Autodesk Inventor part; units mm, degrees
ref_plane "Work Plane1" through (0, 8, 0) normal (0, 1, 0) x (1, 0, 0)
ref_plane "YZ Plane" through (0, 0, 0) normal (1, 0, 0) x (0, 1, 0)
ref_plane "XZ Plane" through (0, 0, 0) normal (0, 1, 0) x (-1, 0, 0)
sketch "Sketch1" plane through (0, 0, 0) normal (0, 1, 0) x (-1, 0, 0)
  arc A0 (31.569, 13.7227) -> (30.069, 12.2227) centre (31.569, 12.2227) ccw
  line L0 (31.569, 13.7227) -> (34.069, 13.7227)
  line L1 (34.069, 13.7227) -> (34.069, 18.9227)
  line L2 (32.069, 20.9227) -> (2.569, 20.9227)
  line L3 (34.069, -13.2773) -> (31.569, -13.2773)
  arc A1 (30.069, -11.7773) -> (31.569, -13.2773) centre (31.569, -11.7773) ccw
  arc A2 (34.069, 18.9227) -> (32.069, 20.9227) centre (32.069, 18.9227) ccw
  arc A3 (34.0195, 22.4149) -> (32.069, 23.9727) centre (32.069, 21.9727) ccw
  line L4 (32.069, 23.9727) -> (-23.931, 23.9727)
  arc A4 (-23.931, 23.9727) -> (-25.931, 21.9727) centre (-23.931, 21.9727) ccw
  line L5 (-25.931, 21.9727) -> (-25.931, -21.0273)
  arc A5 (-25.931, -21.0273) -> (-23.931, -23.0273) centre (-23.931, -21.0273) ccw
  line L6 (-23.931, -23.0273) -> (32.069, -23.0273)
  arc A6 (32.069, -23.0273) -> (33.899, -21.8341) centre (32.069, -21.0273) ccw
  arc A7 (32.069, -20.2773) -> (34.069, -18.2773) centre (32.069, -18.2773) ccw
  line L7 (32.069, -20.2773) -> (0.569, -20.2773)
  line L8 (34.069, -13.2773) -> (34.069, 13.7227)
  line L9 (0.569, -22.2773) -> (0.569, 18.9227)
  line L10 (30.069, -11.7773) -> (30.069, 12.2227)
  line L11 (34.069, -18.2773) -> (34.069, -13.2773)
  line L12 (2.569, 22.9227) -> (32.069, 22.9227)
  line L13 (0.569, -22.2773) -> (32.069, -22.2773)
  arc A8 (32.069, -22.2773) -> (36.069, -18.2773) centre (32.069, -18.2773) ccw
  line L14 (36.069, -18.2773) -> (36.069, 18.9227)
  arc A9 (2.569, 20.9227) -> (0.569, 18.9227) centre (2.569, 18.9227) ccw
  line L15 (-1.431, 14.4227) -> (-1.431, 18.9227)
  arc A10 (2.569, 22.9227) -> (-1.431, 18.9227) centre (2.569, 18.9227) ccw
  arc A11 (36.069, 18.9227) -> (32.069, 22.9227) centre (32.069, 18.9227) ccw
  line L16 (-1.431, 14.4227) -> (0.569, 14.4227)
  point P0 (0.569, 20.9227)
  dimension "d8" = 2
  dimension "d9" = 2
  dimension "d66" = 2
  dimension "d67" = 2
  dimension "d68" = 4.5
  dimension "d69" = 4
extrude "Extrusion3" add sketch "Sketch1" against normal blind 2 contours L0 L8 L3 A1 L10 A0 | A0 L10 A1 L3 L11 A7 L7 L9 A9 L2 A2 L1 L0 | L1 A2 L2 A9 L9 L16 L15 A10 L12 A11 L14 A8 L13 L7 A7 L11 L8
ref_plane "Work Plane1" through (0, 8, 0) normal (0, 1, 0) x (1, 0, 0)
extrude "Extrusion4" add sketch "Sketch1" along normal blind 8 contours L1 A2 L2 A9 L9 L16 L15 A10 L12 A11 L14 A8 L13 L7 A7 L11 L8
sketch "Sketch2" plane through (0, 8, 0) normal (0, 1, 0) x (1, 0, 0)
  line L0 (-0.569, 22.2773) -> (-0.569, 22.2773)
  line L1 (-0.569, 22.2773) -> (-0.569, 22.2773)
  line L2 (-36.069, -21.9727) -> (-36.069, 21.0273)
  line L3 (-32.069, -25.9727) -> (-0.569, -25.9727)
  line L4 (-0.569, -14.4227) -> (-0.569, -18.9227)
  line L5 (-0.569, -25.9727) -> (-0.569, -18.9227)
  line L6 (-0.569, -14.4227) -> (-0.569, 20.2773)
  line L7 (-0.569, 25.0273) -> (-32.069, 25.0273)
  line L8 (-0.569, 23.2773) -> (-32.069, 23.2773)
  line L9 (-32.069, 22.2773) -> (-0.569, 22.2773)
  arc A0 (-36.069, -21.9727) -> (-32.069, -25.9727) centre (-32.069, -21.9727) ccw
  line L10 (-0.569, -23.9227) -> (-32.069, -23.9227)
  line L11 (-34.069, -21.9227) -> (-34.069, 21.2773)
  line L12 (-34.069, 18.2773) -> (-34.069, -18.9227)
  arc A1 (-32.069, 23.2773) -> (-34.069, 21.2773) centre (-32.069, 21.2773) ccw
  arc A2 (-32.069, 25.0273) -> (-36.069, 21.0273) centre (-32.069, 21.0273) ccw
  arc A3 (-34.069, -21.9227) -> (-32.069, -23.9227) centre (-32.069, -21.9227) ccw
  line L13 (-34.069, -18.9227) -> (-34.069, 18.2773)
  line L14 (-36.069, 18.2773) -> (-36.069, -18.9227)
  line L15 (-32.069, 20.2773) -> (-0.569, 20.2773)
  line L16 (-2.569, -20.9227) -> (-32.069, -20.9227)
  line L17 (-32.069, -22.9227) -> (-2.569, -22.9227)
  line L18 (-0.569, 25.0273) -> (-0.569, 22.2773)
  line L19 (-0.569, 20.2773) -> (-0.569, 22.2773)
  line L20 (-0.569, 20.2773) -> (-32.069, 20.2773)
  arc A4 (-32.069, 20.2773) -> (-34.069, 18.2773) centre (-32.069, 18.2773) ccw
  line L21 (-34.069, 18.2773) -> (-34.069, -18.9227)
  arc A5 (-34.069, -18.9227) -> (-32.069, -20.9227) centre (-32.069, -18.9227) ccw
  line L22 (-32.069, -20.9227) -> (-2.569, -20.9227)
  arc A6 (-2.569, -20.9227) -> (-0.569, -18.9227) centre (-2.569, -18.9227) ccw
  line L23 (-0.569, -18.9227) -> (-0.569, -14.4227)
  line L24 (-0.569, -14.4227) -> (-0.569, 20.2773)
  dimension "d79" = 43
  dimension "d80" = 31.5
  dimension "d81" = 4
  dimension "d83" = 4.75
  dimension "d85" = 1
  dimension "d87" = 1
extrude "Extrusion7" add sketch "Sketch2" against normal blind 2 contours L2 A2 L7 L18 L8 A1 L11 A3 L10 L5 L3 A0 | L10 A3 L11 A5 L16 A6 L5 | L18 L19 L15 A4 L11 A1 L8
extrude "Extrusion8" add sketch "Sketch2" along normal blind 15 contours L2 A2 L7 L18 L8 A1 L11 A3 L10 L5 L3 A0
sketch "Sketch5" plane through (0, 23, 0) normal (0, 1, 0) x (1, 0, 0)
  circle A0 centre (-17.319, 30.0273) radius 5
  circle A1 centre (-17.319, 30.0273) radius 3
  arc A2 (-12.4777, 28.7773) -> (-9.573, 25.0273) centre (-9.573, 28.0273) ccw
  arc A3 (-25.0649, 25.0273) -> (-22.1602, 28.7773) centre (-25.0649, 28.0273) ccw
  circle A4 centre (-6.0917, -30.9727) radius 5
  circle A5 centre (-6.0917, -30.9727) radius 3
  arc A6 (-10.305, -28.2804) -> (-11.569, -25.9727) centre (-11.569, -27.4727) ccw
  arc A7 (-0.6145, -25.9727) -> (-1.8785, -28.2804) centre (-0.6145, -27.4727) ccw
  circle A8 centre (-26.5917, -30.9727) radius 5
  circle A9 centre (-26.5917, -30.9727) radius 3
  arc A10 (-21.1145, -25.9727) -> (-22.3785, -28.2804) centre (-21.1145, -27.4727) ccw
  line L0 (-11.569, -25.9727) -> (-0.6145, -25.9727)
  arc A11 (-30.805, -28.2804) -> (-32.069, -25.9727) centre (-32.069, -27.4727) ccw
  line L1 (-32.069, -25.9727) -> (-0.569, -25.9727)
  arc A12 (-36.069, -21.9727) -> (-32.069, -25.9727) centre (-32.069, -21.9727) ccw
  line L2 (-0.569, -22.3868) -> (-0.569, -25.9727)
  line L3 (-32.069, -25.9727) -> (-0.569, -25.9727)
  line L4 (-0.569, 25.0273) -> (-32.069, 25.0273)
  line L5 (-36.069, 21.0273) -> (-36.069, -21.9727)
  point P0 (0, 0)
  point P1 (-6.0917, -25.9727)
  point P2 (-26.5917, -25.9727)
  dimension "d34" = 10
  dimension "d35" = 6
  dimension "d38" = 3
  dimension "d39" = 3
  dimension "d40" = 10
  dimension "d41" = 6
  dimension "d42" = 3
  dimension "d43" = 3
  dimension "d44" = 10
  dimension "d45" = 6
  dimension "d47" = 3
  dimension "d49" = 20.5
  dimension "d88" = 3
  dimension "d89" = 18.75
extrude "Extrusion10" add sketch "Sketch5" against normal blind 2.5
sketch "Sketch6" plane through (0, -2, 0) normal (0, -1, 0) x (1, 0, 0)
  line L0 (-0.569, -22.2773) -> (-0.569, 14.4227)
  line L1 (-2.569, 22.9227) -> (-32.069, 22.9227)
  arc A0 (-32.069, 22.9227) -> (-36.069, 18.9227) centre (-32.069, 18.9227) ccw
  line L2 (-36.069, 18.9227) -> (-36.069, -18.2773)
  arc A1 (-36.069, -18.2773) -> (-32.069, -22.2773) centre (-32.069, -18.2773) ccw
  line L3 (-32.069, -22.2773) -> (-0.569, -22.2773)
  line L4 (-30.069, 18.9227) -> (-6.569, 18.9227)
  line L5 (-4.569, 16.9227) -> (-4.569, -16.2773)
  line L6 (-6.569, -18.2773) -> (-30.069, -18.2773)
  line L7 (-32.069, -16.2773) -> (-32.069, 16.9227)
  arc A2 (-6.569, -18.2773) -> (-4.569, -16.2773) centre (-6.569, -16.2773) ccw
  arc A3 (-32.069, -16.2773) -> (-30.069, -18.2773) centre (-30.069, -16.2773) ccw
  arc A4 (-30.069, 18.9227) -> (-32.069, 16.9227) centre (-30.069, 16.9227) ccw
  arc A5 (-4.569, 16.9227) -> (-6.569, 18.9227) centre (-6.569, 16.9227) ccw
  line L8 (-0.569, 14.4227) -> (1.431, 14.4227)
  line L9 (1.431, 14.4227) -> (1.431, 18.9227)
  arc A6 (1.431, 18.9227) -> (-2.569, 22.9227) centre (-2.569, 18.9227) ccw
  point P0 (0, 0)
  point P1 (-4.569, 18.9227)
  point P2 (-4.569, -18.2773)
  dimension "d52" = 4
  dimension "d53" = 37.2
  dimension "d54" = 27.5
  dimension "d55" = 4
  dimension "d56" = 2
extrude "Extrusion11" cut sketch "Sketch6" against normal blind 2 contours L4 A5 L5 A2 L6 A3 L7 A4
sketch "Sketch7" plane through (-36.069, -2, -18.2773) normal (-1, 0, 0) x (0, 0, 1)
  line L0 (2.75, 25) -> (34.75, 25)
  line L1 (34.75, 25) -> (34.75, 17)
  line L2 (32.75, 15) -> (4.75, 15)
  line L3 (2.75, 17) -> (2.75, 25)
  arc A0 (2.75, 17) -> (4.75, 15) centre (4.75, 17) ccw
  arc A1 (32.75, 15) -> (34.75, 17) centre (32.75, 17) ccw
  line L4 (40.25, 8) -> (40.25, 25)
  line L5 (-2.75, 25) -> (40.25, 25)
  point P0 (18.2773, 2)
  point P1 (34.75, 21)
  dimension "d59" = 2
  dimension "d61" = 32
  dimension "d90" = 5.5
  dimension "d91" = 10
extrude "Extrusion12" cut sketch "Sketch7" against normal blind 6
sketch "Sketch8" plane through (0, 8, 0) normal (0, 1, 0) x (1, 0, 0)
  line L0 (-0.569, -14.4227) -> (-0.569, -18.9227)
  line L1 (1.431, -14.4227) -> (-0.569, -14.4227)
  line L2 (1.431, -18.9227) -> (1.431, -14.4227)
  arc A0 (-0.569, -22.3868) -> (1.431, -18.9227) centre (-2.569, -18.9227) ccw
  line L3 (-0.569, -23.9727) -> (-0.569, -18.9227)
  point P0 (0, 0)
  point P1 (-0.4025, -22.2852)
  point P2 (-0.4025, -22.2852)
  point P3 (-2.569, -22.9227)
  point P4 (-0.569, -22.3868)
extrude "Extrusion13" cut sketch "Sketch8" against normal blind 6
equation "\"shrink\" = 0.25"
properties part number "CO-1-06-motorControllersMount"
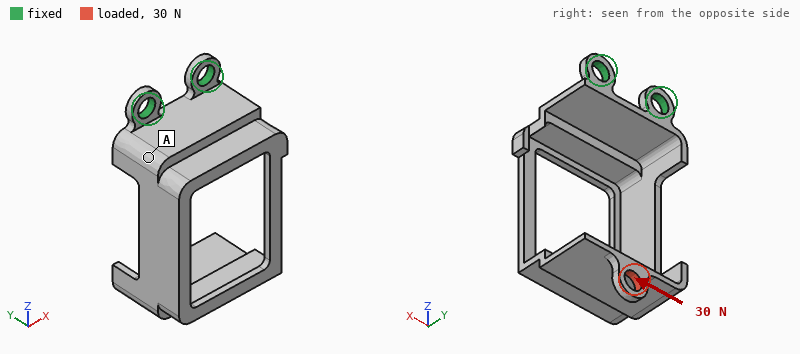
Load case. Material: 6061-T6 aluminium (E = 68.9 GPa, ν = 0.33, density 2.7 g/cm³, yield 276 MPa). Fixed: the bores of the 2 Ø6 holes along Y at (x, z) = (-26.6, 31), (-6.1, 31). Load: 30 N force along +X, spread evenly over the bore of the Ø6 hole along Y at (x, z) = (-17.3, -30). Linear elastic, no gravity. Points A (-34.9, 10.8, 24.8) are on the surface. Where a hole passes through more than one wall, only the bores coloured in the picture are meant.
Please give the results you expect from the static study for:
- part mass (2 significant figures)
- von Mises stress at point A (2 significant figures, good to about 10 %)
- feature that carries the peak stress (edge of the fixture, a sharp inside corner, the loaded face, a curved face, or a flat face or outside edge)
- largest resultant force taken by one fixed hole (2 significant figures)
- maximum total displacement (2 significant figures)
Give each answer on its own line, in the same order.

18 g
22 MPa
a curved face
61 N
0.82 mm
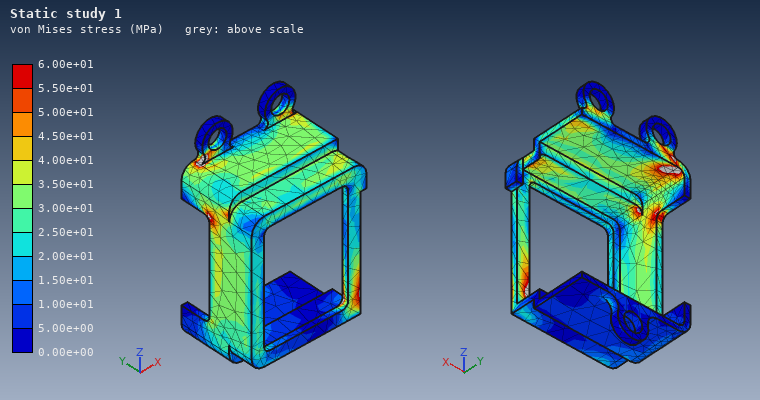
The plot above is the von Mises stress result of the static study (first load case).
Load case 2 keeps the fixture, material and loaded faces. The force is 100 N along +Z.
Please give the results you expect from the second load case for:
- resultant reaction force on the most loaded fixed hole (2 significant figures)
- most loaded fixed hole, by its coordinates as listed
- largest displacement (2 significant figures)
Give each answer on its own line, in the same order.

61 N
(-6.1, 31)
0.95 mm
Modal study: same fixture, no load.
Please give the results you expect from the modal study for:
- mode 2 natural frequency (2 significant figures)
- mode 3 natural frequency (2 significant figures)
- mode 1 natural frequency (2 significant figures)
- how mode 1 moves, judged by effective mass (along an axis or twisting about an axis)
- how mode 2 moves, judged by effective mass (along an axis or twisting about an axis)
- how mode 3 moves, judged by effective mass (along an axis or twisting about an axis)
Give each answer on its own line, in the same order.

490 Hz
1200 Hz
370 Hz
along Y
along X
along Z
